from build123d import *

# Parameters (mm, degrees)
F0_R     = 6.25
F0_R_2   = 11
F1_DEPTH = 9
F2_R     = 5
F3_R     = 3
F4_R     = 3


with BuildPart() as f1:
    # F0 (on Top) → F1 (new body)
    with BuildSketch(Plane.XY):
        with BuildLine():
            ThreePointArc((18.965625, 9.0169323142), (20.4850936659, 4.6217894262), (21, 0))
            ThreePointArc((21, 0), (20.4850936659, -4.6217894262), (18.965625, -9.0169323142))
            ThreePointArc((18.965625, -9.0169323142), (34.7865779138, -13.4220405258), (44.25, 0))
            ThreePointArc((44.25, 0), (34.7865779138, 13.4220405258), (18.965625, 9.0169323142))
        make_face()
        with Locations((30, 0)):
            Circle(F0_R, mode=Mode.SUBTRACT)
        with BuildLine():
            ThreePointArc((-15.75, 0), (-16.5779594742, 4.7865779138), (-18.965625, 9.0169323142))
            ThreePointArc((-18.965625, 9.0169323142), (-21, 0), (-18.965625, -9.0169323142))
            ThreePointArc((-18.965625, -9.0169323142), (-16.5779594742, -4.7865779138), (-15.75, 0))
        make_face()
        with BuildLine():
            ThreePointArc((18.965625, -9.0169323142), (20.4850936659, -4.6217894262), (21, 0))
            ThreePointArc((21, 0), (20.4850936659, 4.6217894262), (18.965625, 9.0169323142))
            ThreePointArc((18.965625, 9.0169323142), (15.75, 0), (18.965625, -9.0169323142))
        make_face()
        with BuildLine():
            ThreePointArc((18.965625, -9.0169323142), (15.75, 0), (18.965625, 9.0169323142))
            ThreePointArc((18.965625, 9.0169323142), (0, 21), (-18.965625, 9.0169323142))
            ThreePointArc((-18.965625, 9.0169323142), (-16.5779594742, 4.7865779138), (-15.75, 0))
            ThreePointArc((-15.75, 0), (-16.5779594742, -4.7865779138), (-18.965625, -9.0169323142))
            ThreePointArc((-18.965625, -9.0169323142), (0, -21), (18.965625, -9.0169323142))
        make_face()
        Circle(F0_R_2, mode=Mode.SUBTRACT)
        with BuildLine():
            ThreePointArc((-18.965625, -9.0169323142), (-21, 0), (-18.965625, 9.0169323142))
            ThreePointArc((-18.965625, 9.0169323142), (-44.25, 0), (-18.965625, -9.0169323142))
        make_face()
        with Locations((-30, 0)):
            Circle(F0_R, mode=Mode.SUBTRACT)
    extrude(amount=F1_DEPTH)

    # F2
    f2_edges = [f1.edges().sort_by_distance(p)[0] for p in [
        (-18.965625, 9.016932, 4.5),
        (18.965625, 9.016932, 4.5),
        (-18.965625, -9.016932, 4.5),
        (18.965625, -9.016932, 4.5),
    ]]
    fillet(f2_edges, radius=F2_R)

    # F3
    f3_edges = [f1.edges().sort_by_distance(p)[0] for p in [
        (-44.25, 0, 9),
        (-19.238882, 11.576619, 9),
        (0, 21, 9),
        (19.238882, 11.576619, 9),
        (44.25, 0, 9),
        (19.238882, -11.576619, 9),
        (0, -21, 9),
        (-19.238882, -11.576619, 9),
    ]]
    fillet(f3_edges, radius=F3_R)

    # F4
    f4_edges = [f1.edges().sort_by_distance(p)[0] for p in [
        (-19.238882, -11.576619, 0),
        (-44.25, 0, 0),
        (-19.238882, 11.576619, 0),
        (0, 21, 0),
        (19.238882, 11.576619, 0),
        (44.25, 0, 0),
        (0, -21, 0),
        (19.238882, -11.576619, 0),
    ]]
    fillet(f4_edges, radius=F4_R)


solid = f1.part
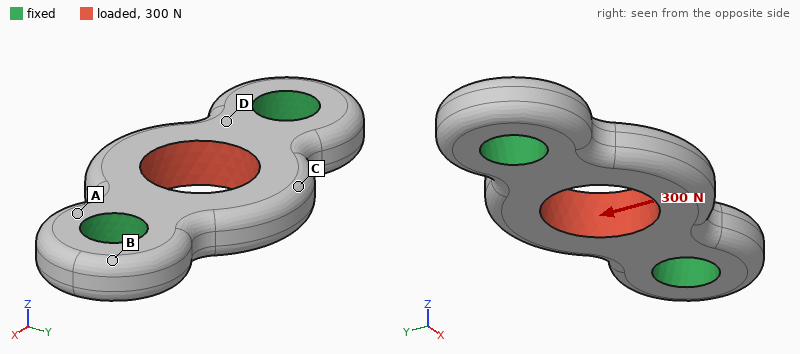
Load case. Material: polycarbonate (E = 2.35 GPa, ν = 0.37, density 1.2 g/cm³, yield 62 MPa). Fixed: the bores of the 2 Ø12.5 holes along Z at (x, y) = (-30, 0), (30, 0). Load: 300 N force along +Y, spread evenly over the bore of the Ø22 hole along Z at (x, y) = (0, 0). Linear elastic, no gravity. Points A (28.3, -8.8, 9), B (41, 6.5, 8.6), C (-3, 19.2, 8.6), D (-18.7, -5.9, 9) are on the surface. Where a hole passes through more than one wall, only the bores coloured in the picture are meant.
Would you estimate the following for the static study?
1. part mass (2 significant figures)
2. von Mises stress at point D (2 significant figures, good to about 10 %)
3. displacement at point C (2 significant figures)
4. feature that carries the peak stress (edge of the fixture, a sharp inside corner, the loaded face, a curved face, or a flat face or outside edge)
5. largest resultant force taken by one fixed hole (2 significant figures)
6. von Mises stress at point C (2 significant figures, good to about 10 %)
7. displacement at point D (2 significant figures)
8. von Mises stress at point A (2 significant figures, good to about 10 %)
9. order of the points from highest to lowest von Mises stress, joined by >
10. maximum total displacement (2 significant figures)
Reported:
20 g
1.4 MPa
19 µm
edge of the fixture
150 N
0.87 MPa
8.1 µm
0.55 MPa
D > C > A > B
21 µm
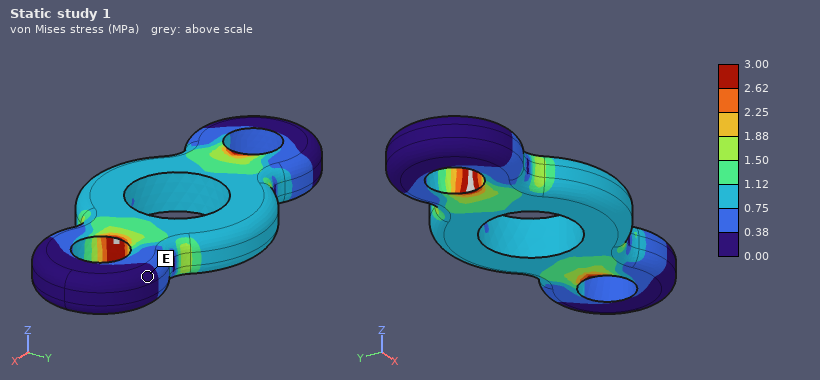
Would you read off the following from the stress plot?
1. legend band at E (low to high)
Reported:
0.00 to 0.38 MPa
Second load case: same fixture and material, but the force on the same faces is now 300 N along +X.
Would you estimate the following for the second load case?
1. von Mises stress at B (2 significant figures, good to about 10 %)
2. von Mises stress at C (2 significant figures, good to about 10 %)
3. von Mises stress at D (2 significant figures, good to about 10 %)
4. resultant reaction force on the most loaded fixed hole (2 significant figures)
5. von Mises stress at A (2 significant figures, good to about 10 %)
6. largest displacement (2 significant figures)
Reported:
0.11 MPa
0.14 MPa
0.68 MPa
150 N
0.40 MPa
9.1 µm
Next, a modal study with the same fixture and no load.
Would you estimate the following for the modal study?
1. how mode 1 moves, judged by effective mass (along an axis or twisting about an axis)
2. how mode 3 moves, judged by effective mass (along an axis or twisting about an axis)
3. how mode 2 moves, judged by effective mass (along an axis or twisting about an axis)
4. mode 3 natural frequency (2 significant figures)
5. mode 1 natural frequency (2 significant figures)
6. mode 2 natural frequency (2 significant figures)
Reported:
twisting about X
along Y
along Z
7100 Hz
3200 Hz
3500 Hz
